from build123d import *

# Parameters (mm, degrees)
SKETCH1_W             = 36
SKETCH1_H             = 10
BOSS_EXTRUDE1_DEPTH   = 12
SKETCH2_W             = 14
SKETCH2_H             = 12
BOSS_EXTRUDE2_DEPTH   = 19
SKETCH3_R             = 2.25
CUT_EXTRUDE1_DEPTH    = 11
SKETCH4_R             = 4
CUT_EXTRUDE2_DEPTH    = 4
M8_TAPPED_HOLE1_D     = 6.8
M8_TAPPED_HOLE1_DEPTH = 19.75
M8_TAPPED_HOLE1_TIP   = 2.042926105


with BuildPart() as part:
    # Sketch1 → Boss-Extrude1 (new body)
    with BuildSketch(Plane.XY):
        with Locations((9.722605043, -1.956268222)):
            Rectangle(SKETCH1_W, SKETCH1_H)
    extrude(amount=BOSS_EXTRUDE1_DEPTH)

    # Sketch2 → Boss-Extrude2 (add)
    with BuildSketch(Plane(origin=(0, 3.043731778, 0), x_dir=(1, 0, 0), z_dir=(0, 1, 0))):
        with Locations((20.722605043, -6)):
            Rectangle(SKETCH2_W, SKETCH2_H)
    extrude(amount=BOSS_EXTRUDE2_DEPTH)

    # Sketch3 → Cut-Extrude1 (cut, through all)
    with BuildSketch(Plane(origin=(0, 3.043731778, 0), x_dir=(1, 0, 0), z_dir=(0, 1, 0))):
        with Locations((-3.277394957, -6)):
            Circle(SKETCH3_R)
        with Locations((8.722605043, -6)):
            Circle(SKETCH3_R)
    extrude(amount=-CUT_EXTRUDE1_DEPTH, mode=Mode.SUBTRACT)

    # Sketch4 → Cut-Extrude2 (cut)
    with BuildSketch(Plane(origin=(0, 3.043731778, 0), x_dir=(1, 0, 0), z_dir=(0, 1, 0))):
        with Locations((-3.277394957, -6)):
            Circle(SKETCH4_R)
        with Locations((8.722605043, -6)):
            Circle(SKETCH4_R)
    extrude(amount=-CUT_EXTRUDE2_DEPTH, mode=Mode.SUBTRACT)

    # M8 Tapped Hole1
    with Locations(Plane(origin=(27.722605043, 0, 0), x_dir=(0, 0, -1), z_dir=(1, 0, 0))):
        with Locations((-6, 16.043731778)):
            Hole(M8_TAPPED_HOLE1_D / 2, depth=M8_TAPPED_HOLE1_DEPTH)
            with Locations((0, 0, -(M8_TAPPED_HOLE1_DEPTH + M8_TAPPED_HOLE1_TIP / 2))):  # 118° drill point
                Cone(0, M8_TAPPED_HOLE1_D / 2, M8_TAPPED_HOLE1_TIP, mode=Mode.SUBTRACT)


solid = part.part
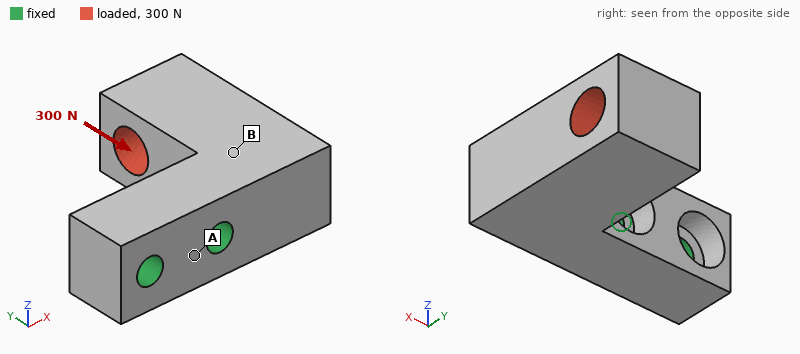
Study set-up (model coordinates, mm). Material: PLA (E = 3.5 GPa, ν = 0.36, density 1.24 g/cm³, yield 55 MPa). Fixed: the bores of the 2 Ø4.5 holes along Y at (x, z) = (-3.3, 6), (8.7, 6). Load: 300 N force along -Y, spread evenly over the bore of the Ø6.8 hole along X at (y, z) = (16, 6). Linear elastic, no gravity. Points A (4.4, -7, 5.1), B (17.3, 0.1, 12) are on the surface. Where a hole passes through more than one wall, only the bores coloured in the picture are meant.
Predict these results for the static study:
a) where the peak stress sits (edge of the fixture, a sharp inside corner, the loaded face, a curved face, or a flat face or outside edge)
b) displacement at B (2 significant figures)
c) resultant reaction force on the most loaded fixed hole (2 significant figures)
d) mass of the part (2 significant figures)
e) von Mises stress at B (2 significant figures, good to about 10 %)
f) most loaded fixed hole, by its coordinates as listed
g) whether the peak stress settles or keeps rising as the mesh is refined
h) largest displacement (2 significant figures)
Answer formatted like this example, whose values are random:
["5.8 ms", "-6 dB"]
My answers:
["edge of the fixture", "0.085 mm", "410 N", "7.9 g", "6.5 MPa", "(8.7, 6)", "keeps rising", "0.36 mm"]
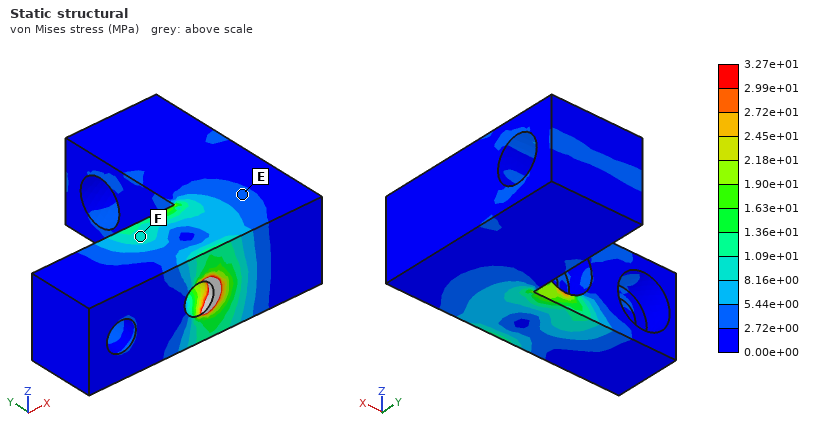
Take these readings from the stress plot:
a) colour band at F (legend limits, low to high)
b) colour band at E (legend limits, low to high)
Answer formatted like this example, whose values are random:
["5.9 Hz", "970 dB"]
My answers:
["8.16e+00 to 1.09e+01 MPa", "2.72e+00 to 5.44e+00 MPa"]
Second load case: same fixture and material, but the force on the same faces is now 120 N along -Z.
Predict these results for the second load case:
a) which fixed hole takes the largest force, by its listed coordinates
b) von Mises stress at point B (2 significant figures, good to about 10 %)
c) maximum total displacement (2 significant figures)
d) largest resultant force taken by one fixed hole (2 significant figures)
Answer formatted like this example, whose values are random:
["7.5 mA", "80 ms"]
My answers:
["(8.7, 6)", "5.8 MPa", "0.36 mm", "170 N"]
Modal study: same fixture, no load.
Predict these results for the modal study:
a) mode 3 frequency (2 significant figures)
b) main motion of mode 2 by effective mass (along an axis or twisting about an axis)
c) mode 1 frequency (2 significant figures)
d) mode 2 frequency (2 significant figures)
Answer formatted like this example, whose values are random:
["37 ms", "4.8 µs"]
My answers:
["4700 Hz", "along Z", "2000 Hz", "2100 Hz"]
